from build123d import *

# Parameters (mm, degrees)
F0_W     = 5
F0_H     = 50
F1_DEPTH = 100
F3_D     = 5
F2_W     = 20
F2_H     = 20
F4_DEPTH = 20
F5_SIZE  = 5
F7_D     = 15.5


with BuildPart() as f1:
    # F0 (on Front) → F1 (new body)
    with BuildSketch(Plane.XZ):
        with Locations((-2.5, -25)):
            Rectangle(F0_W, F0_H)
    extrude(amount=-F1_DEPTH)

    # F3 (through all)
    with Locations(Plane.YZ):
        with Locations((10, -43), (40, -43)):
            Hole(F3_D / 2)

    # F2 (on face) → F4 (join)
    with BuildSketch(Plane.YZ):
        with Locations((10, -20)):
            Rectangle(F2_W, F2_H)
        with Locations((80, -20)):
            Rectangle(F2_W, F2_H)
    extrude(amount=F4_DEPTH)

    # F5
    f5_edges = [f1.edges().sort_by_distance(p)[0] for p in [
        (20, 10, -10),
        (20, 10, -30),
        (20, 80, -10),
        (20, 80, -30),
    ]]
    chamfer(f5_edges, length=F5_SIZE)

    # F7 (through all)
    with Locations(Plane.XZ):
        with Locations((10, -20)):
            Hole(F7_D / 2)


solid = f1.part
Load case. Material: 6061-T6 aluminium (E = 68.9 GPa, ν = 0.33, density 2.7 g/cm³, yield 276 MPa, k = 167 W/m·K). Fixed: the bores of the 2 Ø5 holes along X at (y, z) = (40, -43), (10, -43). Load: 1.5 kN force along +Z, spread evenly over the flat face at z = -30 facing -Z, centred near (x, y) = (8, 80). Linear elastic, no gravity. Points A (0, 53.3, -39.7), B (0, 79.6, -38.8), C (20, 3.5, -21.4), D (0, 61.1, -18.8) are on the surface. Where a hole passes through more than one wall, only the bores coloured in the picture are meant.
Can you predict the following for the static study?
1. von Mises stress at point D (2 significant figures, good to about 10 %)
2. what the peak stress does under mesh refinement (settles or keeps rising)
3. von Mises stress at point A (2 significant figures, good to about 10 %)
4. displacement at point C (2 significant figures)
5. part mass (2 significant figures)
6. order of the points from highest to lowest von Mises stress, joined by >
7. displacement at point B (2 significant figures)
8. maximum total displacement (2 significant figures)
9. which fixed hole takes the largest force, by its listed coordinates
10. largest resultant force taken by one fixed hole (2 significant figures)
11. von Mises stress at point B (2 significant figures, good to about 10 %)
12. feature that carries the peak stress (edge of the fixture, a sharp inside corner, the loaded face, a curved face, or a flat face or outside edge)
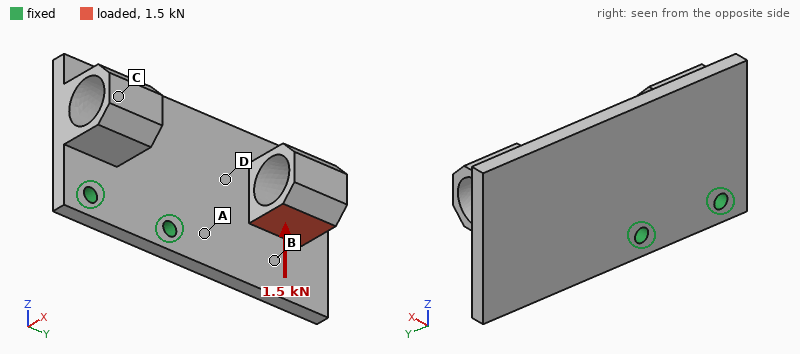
56 MPa
keeps rising
84 MPa
0.078 mm
87 g
A > D > B > C
0.079 mm
0.50 mm
(40, -43)
3.3 kN
42 MPa
edge of the fixture
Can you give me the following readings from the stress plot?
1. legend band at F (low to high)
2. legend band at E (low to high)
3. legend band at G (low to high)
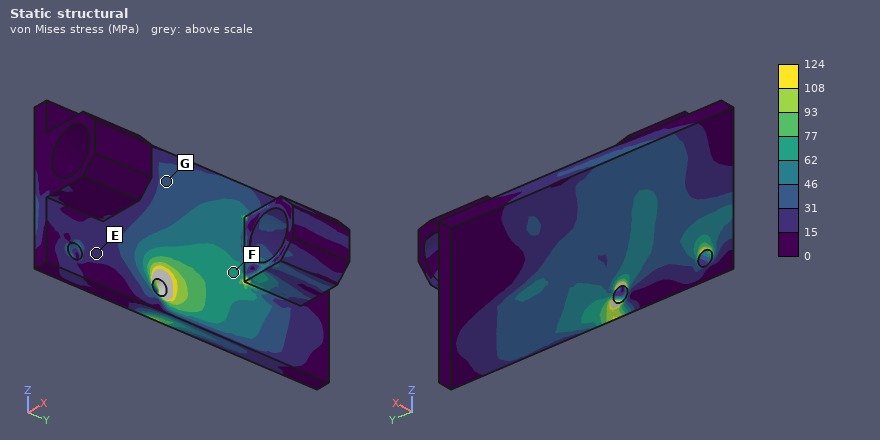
62 to 77 MPa
15 to 31 MPa
31 to 46 MPa
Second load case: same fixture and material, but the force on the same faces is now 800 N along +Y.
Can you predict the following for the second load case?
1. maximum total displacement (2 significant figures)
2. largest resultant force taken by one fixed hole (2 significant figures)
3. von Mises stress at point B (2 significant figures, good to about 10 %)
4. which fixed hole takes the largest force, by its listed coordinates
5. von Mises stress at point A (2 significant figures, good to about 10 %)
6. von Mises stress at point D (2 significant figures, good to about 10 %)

0.41 mm
670 N
15 MPa
(40, -43)
45 MPa
40 MPa
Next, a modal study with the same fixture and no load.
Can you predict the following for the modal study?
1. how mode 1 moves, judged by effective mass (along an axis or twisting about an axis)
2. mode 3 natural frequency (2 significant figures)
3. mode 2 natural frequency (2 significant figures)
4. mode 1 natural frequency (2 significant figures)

along X
2700 Hz
1600 Hz
770 Hz
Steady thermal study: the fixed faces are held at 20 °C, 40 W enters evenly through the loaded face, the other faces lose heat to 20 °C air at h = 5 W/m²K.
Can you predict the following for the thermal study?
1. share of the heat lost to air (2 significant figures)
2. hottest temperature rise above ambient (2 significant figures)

4.9 %
67 K
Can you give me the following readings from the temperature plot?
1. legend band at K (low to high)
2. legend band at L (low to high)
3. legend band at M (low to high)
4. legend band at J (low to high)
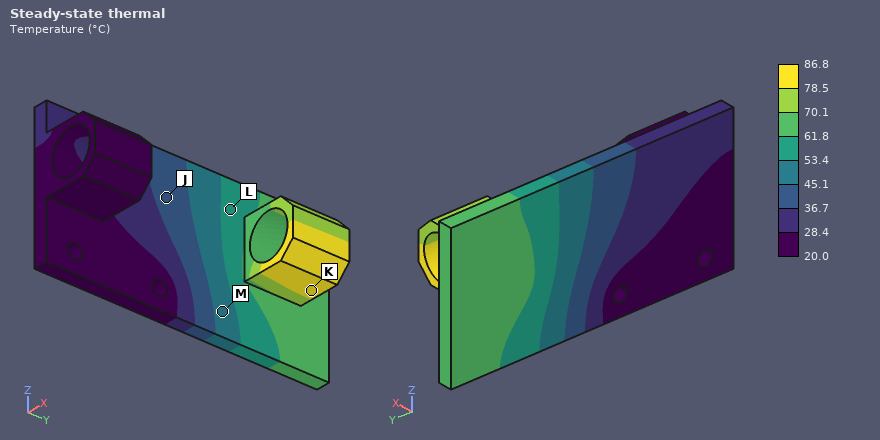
78.5 to 86.8 °C
53.4 to 61.8 °C
45.1 to 53.4 °C
36.7 to 45.1 °C
